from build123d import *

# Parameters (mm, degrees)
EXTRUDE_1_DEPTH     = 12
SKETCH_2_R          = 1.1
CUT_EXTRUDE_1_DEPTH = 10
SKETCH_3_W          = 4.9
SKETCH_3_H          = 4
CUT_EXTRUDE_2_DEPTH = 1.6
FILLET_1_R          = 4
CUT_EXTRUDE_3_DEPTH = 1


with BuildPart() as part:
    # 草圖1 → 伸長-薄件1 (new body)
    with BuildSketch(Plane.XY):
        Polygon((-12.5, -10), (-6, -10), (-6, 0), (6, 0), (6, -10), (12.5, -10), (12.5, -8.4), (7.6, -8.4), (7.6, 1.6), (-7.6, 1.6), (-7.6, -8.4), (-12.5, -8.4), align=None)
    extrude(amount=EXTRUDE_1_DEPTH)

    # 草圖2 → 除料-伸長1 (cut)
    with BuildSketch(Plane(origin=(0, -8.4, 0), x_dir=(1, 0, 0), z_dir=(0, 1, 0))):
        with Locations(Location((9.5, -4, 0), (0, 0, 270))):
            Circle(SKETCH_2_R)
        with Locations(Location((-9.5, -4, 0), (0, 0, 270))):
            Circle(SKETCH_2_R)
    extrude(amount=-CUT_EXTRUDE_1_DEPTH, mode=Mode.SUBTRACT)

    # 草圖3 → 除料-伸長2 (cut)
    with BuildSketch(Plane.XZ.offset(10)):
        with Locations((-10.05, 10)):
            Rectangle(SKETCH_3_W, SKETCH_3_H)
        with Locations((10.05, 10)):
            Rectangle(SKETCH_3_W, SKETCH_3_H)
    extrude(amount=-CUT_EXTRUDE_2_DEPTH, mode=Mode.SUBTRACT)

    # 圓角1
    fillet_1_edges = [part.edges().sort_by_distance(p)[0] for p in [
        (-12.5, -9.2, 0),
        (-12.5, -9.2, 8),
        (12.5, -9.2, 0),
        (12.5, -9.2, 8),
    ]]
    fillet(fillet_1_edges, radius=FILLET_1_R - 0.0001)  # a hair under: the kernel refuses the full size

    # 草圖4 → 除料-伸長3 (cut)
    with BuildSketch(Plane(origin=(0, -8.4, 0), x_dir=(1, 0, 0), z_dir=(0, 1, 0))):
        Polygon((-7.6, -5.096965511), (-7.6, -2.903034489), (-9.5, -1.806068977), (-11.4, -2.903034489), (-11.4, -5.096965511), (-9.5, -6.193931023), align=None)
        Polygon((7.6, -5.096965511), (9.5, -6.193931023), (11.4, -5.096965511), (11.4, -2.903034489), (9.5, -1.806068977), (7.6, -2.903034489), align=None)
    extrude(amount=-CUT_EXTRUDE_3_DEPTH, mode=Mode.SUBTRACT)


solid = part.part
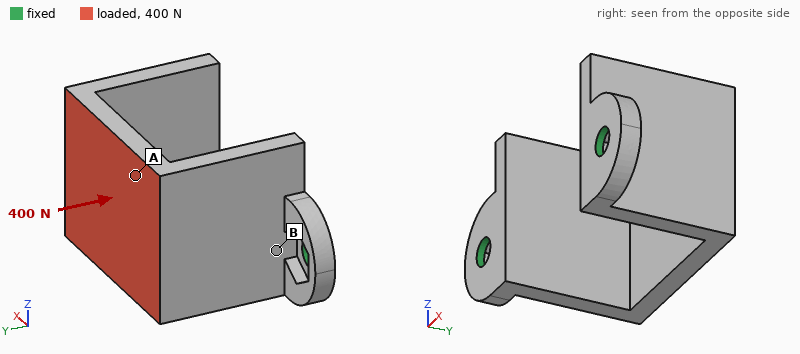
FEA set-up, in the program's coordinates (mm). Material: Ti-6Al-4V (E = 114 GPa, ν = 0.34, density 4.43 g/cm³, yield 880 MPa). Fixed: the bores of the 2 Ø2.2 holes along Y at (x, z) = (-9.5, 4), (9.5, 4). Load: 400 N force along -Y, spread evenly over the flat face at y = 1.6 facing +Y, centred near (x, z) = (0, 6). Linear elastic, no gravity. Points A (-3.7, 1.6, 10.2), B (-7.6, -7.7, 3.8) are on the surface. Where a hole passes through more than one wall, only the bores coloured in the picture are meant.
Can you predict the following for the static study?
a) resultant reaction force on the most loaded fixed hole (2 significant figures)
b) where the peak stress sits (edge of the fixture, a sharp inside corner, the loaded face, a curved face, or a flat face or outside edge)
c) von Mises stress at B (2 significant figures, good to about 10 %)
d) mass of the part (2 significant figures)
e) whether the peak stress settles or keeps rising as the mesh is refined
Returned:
210 N
edge of the fixture
61 MPa
3.3 g
keeps rising
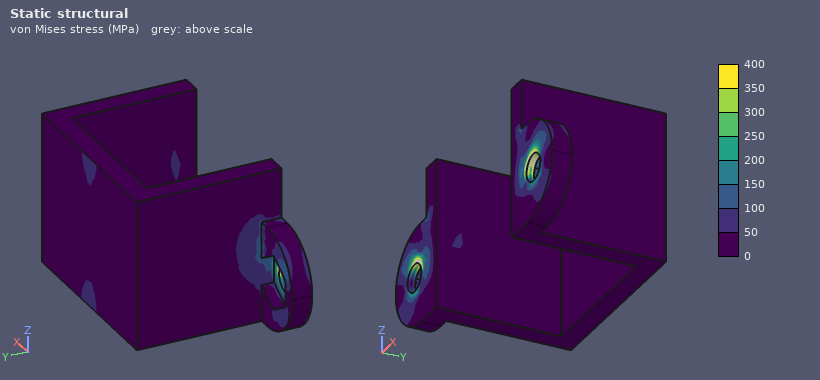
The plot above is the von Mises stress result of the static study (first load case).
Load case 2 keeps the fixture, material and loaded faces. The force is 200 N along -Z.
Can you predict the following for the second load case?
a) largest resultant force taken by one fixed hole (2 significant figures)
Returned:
100 N
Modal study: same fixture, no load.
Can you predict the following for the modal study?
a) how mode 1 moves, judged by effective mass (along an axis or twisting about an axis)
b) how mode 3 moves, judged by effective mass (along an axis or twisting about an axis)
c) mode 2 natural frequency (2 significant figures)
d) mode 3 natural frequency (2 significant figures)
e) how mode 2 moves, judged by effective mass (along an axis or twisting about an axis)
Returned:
along Z
twisting about Y
7200 Hz
9900 Hz
along X
